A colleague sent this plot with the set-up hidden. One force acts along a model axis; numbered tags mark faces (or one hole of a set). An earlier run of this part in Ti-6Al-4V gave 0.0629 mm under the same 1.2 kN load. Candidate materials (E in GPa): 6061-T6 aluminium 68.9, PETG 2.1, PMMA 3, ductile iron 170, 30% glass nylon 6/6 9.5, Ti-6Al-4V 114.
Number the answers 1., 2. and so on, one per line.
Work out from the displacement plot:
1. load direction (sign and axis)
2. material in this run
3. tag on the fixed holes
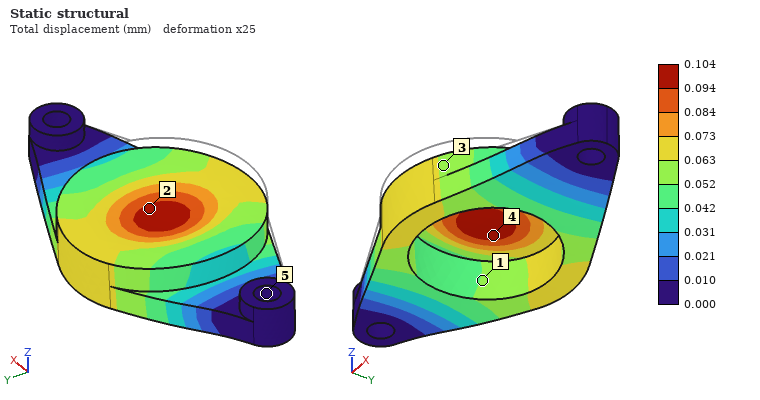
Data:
1. -Z
2. 6061-T6 aluminium
3. 5
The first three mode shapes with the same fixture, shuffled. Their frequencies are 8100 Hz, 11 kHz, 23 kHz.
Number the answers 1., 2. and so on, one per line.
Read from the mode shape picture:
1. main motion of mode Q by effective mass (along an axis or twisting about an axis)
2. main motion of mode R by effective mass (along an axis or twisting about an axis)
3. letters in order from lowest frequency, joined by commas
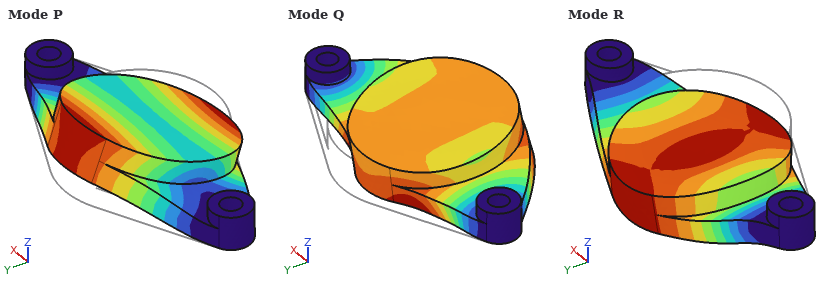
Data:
1. along Y
2. along Z
3. P, R, Q
